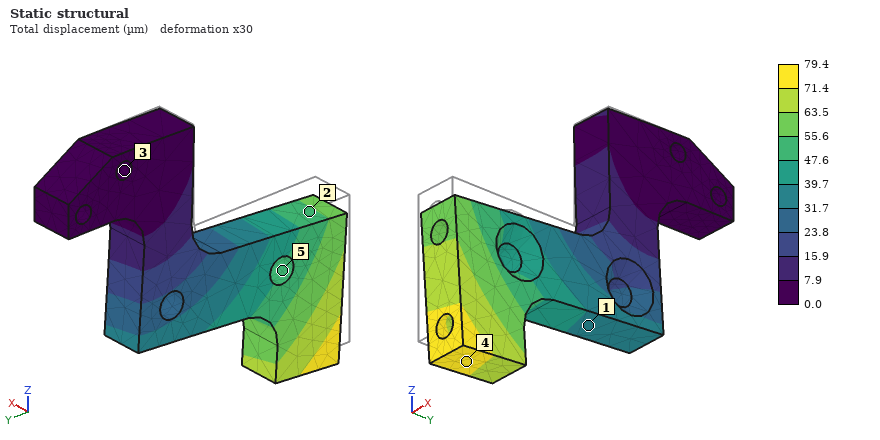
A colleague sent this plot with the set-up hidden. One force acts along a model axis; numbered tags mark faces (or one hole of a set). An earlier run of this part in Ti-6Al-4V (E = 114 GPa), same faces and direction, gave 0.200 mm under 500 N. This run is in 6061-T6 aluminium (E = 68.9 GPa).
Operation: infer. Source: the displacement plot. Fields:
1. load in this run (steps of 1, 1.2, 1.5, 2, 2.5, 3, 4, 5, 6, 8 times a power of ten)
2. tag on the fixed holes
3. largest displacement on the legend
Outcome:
120 N
3
79.4 µm
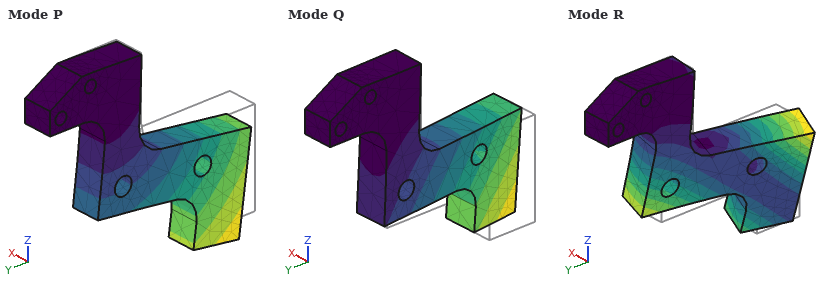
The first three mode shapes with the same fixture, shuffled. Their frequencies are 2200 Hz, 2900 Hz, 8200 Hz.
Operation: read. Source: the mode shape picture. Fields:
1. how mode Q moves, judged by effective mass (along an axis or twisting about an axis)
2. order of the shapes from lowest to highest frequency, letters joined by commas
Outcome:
along X
Q, P, R
